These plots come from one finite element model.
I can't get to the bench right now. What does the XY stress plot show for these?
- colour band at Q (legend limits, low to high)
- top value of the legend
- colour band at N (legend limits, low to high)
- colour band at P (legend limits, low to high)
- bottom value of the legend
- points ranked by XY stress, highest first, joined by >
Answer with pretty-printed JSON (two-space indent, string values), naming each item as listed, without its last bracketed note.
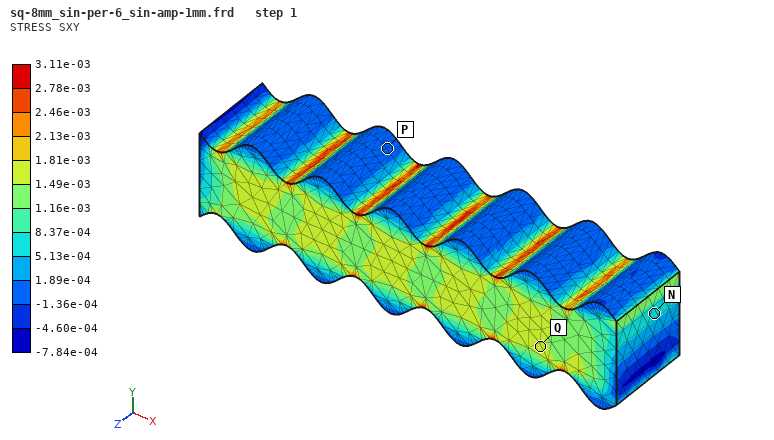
{
  "colour band at Q": "1.49e-03 to 1.81e-03",
  "top value of the legend": "3.11e-03",
  "colour band at N": "5.13e-04 to 8.37e-04",
  "colour band at P": "-1.36e-04 to 1.89e-04",
  "bottom value of the legend": "-7.84e-04",
  "points ranked by XY stress, highest first, joined by >": "Q > N > P"
}
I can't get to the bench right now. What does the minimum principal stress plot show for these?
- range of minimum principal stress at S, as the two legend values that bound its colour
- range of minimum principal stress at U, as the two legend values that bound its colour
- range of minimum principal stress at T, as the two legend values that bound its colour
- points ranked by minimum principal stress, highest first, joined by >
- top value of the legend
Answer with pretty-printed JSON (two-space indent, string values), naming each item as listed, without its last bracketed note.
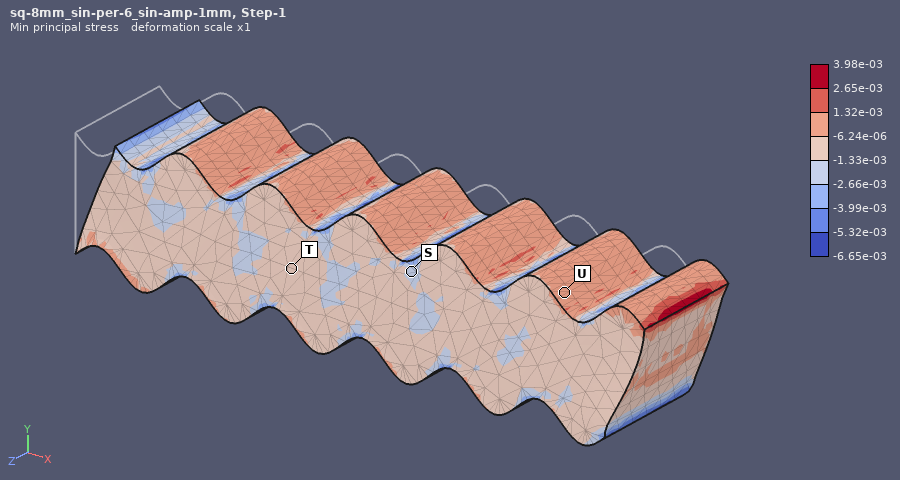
{
  "range of minimum principal stress at S, as the two legend values that bound its colour": "-2.66e-03 to -1.33e-03",
  "range of minimum principal stress at U, as the two legend values that bound its colour": "-6.24e-06 to 1.32e-03",
  "range of minimum principal stress at T, as the two legend values that bound its colour": "-1.33e-03 to -6.24e-06",
  "points ranked by minimum principal stress, highest first, joined by >": "U > T > S",
  "top value of the legend": "3.98e-03"
}
